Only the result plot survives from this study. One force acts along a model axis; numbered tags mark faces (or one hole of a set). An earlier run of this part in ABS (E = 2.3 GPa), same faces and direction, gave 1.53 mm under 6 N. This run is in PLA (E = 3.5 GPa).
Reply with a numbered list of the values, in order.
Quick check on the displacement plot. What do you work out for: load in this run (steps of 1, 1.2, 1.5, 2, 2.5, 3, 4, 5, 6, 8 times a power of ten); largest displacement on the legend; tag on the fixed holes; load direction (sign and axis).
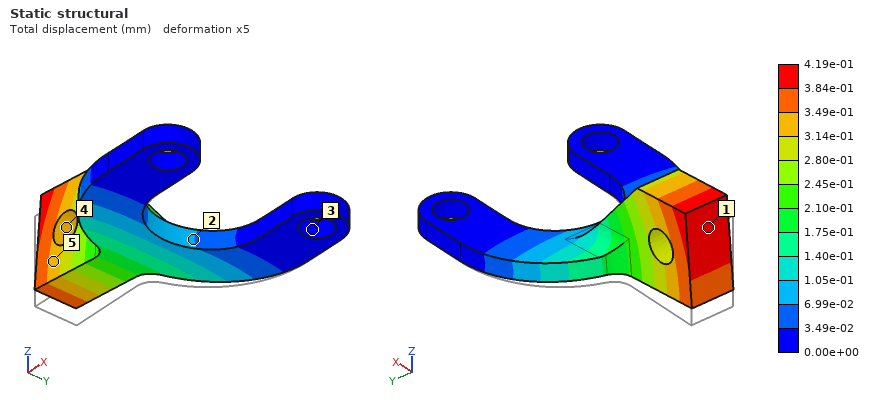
1. 2.5 N
2. 4.19e-01 mm
3. 3
4. +Z
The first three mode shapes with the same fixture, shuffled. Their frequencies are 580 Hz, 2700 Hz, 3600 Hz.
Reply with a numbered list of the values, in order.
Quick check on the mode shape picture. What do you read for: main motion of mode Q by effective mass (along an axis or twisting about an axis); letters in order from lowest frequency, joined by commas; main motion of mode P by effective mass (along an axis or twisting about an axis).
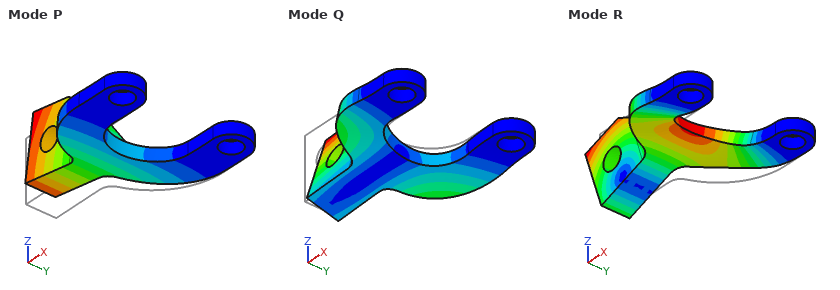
1. along Y
2. P, Q, R
3. along Z
